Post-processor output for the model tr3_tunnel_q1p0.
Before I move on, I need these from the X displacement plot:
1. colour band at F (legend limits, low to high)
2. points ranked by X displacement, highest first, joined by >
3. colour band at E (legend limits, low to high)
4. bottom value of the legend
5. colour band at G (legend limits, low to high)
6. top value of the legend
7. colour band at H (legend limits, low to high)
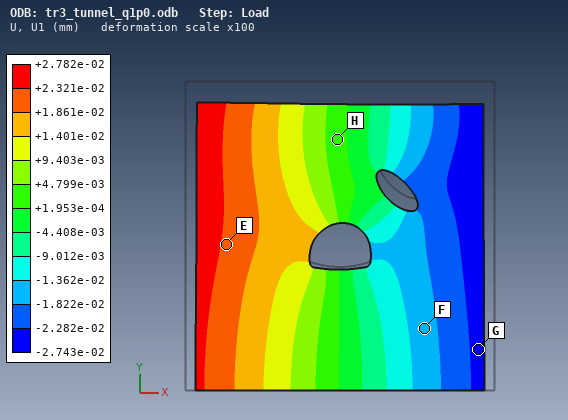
-1.822e-02 to -1.362e-02 mm
E > H > F > G
+1.861e-02 to +2.321e-02 mm
-2.743e-02 mm
-2.743e-02 to -2.282e-02 mm
+2.782e-02 mm
+1.953e-04 to +4.799e-03 mm
